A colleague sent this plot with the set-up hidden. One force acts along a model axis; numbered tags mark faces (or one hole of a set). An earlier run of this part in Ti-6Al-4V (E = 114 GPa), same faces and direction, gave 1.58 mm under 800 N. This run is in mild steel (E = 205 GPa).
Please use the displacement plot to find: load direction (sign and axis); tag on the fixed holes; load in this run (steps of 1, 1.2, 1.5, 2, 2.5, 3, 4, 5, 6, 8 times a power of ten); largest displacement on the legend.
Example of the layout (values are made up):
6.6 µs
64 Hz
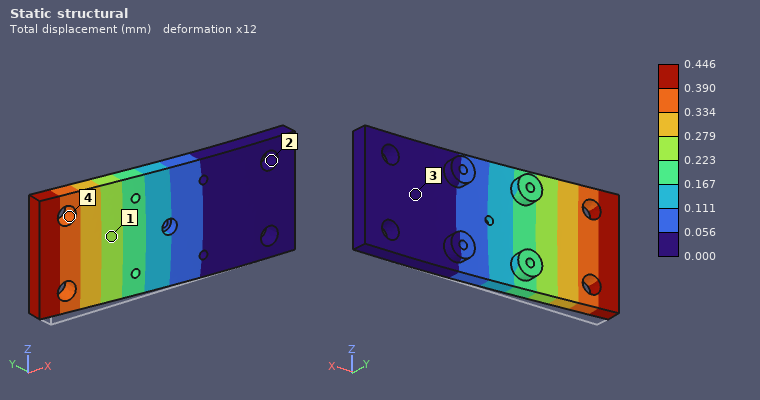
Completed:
+Y
2
400 N
0.446 mm
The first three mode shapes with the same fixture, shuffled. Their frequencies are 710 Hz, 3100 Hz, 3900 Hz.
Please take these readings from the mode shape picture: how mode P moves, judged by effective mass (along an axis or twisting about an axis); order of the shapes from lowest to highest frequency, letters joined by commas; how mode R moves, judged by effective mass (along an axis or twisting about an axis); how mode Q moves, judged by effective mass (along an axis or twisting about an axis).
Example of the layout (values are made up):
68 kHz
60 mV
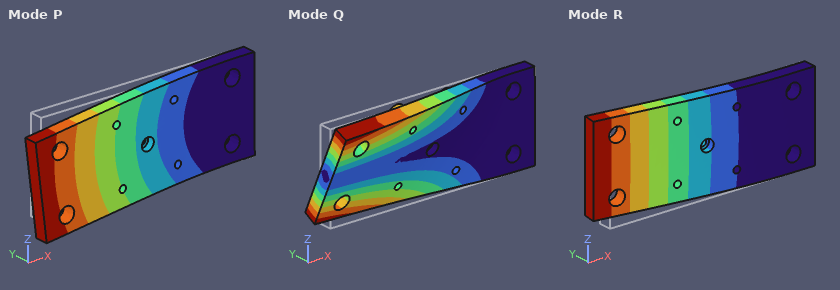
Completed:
along Z
R, Q, P
along Y
twisting about X
